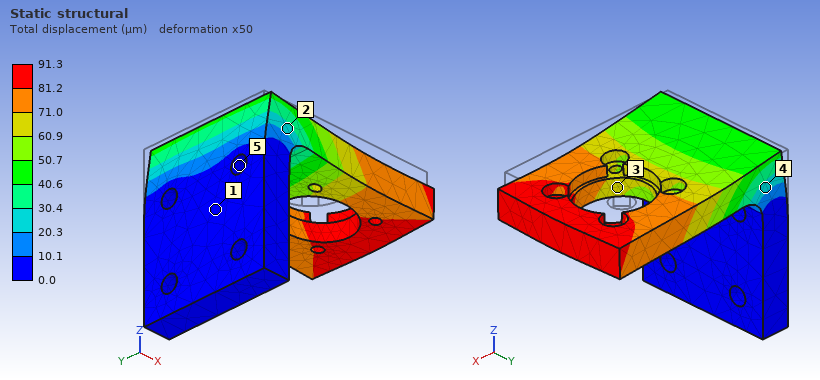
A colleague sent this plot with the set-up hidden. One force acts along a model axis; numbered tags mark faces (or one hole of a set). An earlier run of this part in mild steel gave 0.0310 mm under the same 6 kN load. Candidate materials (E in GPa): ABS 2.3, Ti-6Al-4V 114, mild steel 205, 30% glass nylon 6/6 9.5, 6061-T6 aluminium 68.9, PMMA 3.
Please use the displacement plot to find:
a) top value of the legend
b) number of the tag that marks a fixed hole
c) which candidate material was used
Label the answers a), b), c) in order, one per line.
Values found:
a) 91.3 µm
b) 5
c) 6061-T6 aluminium
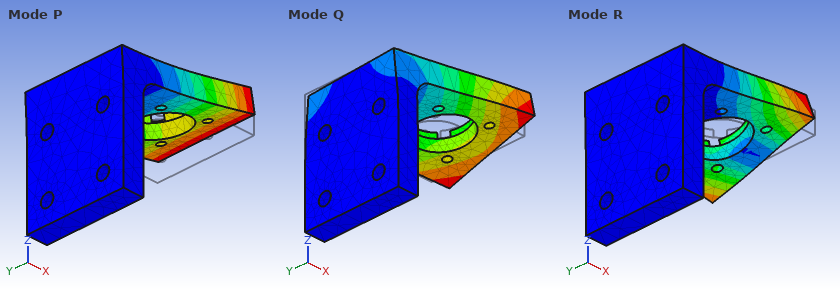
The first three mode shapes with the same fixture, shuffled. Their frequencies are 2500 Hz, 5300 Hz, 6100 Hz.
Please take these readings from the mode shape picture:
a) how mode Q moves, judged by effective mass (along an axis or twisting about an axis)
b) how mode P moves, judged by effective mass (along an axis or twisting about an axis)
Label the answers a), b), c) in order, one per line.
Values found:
a) along Y
b) along Z
